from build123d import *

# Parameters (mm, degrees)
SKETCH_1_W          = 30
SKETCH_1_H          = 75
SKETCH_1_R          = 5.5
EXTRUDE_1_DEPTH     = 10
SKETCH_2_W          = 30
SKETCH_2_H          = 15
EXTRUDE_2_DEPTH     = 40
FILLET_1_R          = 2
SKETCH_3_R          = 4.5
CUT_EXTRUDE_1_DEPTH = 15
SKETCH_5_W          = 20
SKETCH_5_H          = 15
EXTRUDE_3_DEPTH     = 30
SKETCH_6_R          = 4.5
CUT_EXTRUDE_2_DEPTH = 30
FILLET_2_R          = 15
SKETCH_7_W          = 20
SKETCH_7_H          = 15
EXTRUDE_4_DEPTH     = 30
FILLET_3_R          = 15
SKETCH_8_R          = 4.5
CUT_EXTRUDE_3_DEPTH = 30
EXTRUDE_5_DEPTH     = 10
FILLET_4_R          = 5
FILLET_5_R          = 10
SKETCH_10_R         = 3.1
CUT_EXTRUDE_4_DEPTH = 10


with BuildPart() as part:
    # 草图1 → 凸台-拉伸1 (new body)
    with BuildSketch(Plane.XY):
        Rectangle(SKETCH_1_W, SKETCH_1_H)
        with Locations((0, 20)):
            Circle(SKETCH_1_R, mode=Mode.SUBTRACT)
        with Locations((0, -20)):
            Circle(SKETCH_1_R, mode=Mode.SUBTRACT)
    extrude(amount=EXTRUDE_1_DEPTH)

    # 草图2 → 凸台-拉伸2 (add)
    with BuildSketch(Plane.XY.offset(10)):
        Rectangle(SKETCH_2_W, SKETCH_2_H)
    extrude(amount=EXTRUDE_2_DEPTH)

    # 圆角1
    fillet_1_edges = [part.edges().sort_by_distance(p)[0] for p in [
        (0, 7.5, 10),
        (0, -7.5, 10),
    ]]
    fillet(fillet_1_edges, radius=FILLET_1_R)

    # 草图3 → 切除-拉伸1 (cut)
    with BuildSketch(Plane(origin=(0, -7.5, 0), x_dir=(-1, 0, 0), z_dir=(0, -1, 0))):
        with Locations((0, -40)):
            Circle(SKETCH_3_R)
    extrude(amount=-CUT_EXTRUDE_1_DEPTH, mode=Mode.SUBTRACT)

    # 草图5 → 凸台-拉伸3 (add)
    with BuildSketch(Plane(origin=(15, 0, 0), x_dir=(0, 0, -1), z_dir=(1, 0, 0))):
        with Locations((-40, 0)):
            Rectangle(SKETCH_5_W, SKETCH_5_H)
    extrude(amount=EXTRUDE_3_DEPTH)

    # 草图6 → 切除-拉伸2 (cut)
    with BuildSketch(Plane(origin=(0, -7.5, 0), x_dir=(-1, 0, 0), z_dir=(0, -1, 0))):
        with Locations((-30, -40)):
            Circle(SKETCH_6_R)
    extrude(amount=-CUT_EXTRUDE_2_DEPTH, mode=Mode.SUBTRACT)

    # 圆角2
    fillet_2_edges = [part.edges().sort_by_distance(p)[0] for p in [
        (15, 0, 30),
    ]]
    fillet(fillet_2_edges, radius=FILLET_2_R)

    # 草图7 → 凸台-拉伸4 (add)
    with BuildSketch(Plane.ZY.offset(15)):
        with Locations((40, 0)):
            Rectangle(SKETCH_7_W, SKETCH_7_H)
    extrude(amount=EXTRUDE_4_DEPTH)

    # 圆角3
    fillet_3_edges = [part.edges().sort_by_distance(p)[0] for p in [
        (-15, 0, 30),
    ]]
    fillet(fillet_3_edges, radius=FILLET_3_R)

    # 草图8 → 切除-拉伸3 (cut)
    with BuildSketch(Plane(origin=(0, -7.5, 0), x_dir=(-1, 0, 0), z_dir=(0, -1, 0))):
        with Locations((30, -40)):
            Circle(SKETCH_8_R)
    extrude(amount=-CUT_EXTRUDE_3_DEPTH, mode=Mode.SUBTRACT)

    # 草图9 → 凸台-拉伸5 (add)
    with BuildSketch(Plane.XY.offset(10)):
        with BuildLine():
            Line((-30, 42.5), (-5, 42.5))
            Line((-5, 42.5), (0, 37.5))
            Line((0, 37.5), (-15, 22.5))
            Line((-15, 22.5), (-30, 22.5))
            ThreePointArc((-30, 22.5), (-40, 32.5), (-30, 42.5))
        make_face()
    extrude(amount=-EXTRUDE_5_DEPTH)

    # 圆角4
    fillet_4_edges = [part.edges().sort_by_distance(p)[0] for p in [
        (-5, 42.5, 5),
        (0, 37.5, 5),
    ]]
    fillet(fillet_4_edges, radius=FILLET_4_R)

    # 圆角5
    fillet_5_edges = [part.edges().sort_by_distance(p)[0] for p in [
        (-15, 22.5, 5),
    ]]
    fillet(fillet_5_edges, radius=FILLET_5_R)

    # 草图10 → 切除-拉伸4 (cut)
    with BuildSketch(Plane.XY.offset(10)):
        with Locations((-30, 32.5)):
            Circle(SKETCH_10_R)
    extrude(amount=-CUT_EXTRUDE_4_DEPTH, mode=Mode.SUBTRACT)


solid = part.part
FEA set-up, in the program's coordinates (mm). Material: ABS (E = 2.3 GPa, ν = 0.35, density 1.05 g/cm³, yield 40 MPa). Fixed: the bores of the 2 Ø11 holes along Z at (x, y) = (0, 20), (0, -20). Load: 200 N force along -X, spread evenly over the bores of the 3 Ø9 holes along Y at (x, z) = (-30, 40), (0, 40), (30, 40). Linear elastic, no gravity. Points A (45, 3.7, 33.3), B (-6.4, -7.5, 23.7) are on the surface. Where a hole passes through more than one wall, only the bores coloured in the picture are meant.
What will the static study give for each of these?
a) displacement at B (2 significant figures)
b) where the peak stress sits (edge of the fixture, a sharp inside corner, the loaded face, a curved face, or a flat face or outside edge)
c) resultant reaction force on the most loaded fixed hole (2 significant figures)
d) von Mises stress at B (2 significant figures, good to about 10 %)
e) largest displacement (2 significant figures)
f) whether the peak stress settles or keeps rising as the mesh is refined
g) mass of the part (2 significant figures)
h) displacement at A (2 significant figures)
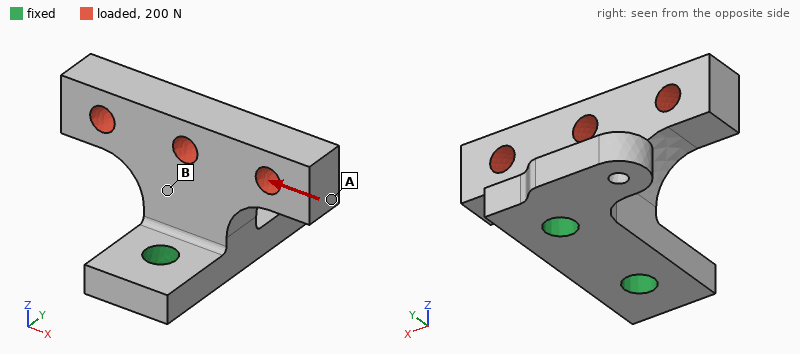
0.10 mm
edge of the fixture
100 N
1.2 MPa
0.35 mm
keeps rising
63 g
0.29 mm
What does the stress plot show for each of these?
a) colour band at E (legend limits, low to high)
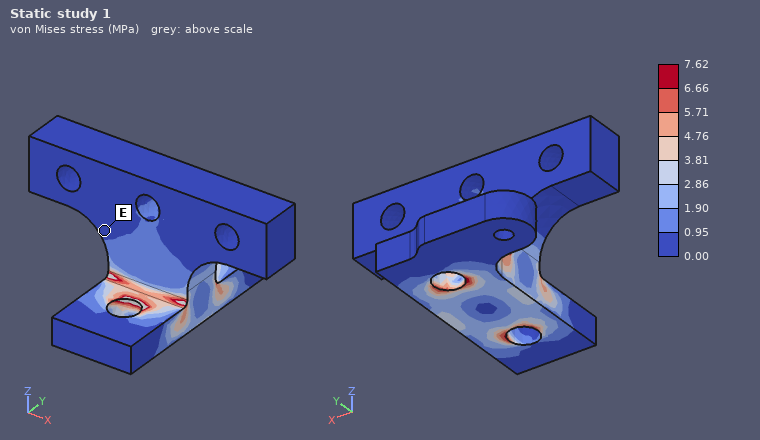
0.00 to 0.95 MPa
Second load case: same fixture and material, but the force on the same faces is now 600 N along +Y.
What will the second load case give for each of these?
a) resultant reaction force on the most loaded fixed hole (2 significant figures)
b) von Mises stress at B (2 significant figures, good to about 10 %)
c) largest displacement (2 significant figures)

800 N
6.8 MPa
0.81 mm
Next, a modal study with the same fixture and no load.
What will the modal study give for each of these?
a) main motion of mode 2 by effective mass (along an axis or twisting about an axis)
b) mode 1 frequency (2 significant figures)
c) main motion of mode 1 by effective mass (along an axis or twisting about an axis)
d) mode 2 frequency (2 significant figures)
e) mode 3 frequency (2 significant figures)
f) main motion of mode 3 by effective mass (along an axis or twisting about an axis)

along Y
770 Hz
along X
1000 Hz
1100 Hz
twisting about Z
